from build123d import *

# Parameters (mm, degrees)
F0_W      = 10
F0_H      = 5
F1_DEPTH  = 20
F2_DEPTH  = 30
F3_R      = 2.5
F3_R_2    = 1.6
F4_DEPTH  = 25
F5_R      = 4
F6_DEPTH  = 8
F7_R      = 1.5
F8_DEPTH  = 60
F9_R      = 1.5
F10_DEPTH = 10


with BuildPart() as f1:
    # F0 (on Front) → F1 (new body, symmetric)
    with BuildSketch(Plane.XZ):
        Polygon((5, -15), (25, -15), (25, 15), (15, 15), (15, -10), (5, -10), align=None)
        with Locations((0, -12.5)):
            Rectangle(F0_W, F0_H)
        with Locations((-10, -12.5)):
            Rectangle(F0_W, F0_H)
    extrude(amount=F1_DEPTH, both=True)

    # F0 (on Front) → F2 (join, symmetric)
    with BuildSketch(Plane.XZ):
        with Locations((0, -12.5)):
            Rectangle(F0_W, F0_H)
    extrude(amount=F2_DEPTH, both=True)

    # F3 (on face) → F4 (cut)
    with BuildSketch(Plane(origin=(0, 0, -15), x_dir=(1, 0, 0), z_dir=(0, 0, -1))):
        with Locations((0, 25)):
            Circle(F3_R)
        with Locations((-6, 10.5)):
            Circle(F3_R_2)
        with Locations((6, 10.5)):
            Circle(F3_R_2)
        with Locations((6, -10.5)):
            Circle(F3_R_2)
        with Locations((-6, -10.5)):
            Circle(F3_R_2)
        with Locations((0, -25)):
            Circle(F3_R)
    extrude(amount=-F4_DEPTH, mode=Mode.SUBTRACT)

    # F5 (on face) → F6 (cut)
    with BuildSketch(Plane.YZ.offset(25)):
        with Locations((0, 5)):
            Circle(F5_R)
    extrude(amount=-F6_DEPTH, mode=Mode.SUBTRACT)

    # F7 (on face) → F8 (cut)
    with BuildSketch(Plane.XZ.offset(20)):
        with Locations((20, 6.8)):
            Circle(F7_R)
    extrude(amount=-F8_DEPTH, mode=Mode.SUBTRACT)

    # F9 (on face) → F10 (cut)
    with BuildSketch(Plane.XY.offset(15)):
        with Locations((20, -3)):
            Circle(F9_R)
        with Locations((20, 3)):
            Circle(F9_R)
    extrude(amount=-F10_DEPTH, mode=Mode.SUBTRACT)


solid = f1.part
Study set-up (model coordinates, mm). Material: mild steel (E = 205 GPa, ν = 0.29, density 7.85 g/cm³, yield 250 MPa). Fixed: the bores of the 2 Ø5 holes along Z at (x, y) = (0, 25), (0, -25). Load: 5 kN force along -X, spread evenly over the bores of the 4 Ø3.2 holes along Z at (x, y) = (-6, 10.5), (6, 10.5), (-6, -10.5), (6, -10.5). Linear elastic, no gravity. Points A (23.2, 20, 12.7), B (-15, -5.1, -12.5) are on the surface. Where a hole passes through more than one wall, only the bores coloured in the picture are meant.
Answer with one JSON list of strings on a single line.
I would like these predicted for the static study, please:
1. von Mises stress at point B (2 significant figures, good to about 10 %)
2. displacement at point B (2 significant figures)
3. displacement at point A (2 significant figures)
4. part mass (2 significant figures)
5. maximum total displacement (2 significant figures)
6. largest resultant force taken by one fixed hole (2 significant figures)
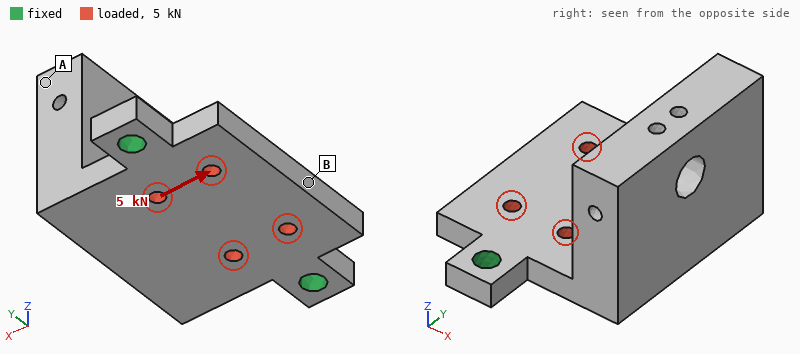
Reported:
["33 MPa", "7.2 µm", "6.9 µm", "140 g", "7.6 µm", "2.5 kN"]
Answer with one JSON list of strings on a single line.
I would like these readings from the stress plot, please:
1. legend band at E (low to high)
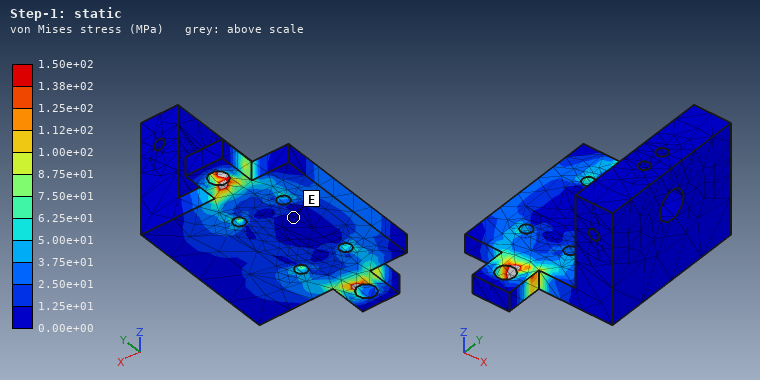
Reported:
["0.00e+00 to 1.25e+01 MPa"]
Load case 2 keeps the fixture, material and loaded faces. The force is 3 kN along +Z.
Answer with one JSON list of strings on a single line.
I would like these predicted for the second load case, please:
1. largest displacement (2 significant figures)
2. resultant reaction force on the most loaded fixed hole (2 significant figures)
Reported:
["32 µm", "1.5 kN"]
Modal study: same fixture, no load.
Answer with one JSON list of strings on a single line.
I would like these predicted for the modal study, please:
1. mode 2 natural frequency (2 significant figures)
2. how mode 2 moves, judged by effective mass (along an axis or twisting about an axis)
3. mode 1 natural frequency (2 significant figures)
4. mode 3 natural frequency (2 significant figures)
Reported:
["3900 Hz", "along Y", "1400 Hz", "5400 Hz"]
